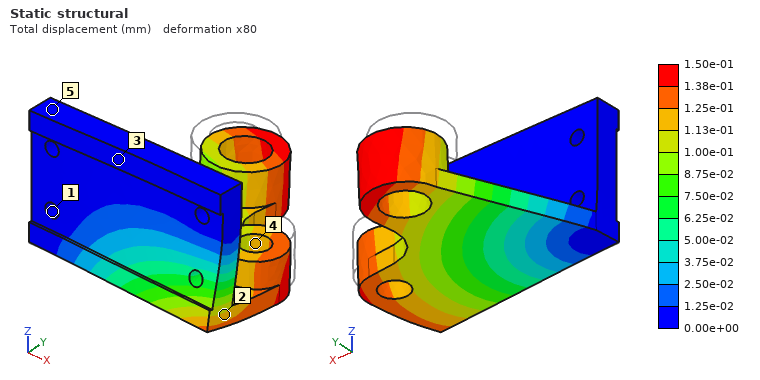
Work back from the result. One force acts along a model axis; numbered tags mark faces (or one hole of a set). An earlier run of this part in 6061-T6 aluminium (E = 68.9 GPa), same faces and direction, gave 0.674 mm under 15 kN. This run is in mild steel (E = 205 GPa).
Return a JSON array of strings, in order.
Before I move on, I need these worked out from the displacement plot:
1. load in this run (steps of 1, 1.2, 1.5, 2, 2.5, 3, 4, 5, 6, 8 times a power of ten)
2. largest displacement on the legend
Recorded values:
["10 kN", "1.50e-01 mm"]
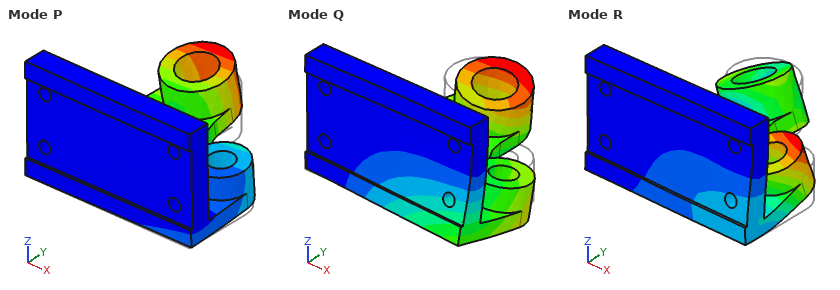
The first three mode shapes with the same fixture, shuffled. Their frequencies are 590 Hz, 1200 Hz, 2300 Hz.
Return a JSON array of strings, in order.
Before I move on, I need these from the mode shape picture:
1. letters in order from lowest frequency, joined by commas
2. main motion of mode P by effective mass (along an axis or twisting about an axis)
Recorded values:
["P, Q, R", "along Z"]
